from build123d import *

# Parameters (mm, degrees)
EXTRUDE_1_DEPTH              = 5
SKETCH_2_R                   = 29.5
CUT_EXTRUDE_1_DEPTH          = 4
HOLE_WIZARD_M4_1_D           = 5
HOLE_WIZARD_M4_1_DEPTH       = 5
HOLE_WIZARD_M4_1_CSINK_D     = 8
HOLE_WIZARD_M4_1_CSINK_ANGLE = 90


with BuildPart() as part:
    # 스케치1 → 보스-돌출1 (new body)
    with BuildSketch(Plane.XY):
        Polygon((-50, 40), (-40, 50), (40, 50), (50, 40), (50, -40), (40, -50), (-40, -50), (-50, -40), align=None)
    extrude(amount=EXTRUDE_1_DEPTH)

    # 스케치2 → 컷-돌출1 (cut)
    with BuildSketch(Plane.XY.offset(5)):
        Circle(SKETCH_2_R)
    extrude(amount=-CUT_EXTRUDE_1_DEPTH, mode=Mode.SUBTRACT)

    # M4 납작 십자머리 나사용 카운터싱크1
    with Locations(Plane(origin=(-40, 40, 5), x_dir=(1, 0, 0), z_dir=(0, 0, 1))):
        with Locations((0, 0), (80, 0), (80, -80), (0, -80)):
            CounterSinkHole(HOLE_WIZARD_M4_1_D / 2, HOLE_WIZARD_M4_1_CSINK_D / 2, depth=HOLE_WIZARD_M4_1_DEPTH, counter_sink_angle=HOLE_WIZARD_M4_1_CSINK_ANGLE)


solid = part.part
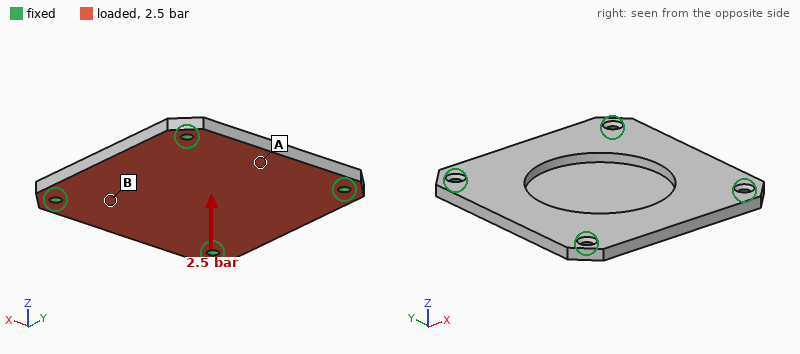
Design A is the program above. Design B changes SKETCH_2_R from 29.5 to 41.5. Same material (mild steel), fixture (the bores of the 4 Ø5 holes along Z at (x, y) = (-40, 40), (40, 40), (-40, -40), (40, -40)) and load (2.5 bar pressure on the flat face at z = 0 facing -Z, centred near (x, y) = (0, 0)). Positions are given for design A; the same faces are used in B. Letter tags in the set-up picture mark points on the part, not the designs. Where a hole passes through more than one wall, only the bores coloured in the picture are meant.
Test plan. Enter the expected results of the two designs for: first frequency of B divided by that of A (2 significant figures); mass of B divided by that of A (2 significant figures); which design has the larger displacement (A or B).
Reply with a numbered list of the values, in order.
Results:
1. 0.56
2. 0.72
3. B
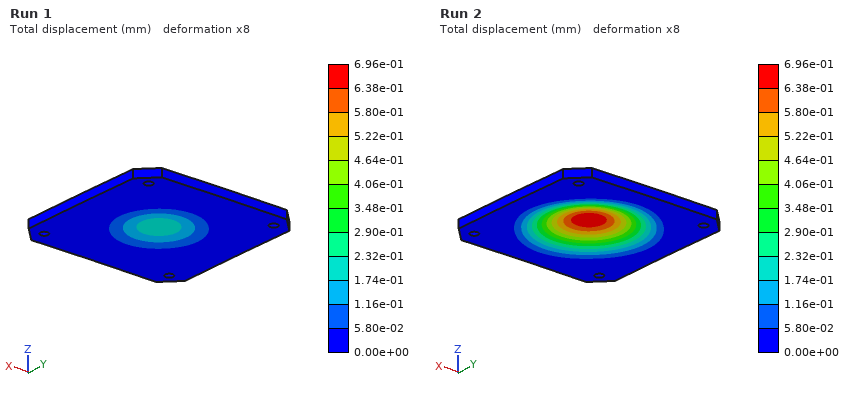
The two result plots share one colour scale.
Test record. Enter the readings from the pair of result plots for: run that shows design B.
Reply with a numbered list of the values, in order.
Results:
1. Run 2
